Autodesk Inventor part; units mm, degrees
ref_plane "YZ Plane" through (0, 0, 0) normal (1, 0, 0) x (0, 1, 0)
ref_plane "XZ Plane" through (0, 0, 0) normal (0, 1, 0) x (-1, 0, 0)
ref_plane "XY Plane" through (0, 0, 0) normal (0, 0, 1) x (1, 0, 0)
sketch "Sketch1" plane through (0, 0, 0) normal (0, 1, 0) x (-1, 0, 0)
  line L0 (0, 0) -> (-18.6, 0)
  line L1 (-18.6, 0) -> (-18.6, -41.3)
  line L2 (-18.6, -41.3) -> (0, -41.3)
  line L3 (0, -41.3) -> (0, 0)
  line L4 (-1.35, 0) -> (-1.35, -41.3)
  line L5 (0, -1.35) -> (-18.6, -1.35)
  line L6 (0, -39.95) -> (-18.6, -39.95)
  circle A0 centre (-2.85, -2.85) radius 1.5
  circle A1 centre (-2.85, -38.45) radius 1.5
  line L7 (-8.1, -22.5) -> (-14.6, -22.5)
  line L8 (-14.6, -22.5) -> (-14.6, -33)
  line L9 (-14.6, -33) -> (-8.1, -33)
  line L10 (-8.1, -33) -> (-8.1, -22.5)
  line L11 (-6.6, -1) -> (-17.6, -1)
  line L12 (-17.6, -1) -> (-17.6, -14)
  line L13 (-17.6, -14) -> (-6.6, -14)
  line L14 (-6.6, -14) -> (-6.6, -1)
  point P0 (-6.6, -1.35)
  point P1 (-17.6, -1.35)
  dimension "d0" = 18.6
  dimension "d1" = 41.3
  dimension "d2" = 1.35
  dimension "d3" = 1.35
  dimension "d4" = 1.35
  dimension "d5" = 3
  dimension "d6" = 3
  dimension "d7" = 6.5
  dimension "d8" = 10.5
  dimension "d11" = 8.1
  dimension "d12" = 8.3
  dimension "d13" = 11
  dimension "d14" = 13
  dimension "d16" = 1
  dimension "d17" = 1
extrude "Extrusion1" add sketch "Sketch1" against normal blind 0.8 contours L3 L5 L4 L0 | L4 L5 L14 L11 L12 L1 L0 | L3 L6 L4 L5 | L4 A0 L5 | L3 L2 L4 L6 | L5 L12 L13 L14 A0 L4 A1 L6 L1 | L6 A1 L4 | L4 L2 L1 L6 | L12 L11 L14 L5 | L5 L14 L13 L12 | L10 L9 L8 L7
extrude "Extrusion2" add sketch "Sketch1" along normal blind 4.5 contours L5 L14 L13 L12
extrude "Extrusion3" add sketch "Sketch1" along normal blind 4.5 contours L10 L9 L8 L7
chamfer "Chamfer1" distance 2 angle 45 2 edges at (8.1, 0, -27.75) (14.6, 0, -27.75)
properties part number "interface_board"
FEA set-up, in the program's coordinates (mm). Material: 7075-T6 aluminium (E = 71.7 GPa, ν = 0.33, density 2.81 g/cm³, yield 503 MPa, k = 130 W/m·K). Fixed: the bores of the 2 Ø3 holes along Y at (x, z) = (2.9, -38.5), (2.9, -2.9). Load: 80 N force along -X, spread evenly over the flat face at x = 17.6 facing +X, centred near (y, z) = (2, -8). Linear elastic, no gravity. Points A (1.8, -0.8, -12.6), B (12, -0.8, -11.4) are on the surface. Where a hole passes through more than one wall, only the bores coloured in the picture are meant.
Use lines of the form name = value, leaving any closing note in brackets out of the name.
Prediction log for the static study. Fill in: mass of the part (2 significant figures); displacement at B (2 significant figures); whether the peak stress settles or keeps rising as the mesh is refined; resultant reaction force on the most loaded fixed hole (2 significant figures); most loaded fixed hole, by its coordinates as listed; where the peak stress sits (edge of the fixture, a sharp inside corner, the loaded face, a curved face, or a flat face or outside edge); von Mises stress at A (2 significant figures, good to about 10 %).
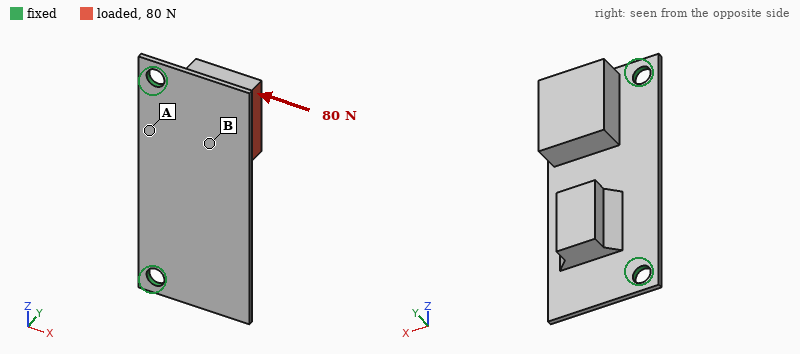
mass of the part = 4.4 g
displacement at B = 0.095 mm
whether the peak stress settles or keeps rising as the mesh is refined = keeps rising
resultant reaction force on the most loaded fixed hole = 71 N
most loaded fixed hole, by its coordinates as listed = (2.9, -2.9)
where the peak stress sits = edge of the fixture
von Mises stress at A = 30 MPa
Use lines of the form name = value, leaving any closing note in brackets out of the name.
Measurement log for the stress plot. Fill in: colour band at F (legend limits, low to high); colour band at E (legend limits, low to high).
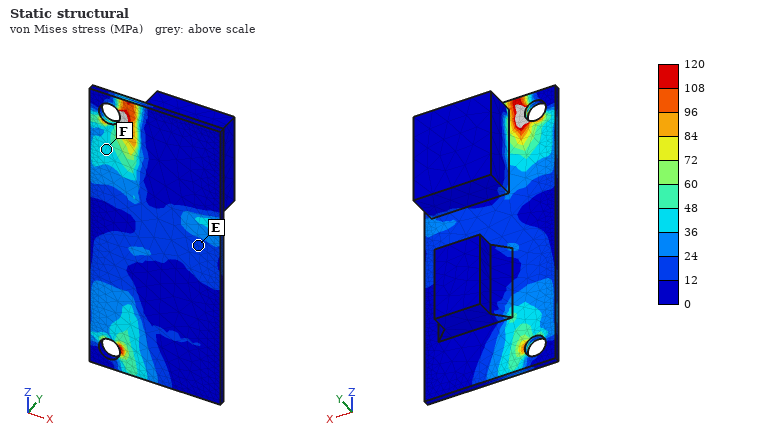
colour band at F = 36 to 48 MPa
colour band at E = 12 to 24 MPa
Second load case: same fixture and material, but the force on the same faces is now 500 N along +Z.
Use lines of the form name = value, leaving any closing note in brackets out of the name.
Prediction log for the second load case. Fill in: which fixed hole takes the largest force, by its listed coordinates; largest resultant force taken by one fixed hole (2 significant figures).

which fixed hole takes the largest force, by its listed coordinates = (2.9, -38.5)
largest resultant force taken by one fixed hole = 350 N
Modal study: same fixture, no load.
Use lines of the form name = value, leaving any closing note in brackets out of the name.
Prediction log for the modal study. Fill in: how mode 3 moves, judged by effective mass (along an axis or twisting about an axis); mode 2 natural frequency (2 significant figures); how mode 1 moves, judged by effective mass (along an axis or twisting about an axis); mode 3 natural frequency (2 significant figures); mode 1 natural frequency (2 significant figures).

how mode 3 moves, judged by effective mass = twisting about X
mode 2 natural frequency = 3400 Hz
how mode 1 moves, judged by effective mass = along Y
mode 3 natural frequency = 3900 Hz
mode 1 natural frequency = 1200 Hz
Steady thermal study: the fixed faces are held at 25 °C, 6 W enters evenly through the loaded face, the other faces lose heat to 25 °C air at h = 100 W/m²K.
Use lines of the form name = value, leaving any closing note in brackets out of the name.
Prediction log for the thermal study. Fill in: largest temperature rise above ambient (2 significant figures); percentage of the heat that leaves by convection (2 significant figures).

largest temperature rise above ambient = 21 K
percentage of the heat that leaves by convection = 31 %
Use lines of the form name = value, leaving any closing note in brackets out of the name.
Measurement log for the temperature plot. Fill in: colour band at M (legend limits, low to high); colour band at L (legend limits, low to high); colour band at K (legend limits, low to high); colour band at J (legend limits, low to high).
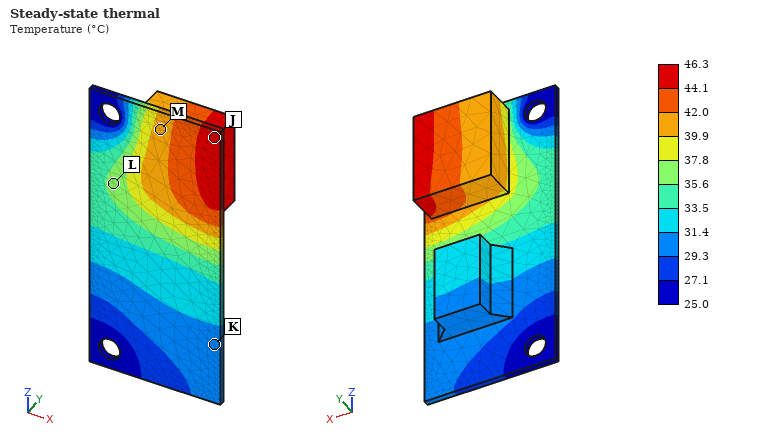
colour band at M = 39.9 to 42.0 °C
colour band at L = 35.6 to 37.8 °C
colour band at K = 29.3 to 31.4 °C
colour band at J = 44.1 to 46.3 °C
